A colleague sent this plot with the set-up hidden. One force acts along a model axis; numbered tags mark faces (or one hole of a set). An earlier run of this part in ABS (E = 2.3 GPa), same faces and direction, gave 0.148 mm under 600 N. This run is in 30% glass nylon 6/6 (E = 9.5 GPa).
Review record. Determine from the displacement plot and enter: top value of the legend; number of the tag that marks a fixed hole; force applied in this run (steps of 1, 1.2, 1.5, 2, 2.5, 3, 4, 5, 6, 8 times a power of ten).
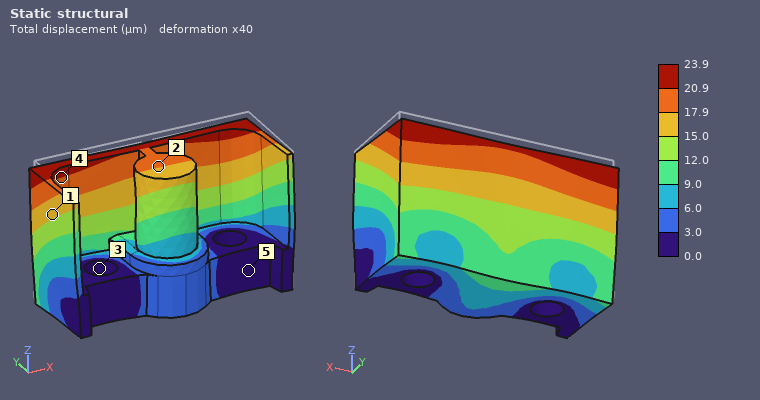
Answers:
23.9 µm
3
400 N
